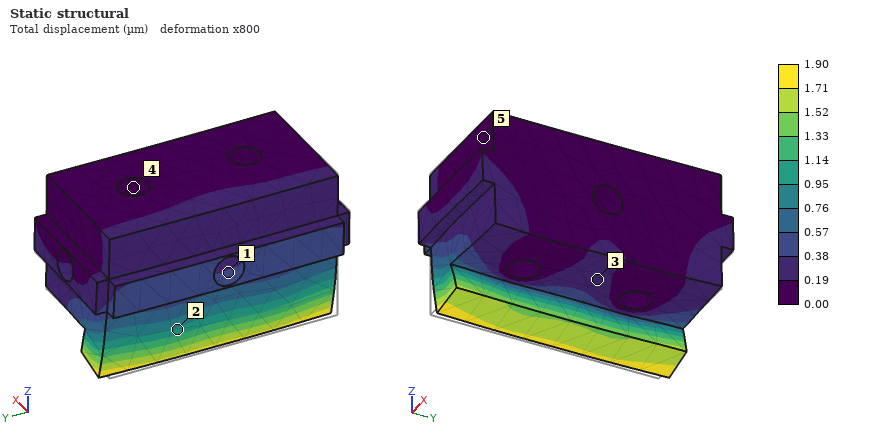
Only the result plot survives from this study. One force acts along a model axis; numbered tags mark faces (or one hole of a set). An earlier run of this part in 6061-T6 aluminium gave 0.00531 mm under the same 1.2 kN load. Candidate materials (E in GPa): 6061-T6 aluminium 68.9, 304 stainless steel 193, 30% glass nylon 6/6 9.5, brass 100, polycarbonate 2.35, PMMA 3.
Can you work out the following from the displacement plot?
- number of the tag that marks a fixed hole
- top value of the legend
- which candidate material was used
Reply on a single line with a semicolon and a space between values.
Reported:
4; 1.90 µm; 304 stainless steel
